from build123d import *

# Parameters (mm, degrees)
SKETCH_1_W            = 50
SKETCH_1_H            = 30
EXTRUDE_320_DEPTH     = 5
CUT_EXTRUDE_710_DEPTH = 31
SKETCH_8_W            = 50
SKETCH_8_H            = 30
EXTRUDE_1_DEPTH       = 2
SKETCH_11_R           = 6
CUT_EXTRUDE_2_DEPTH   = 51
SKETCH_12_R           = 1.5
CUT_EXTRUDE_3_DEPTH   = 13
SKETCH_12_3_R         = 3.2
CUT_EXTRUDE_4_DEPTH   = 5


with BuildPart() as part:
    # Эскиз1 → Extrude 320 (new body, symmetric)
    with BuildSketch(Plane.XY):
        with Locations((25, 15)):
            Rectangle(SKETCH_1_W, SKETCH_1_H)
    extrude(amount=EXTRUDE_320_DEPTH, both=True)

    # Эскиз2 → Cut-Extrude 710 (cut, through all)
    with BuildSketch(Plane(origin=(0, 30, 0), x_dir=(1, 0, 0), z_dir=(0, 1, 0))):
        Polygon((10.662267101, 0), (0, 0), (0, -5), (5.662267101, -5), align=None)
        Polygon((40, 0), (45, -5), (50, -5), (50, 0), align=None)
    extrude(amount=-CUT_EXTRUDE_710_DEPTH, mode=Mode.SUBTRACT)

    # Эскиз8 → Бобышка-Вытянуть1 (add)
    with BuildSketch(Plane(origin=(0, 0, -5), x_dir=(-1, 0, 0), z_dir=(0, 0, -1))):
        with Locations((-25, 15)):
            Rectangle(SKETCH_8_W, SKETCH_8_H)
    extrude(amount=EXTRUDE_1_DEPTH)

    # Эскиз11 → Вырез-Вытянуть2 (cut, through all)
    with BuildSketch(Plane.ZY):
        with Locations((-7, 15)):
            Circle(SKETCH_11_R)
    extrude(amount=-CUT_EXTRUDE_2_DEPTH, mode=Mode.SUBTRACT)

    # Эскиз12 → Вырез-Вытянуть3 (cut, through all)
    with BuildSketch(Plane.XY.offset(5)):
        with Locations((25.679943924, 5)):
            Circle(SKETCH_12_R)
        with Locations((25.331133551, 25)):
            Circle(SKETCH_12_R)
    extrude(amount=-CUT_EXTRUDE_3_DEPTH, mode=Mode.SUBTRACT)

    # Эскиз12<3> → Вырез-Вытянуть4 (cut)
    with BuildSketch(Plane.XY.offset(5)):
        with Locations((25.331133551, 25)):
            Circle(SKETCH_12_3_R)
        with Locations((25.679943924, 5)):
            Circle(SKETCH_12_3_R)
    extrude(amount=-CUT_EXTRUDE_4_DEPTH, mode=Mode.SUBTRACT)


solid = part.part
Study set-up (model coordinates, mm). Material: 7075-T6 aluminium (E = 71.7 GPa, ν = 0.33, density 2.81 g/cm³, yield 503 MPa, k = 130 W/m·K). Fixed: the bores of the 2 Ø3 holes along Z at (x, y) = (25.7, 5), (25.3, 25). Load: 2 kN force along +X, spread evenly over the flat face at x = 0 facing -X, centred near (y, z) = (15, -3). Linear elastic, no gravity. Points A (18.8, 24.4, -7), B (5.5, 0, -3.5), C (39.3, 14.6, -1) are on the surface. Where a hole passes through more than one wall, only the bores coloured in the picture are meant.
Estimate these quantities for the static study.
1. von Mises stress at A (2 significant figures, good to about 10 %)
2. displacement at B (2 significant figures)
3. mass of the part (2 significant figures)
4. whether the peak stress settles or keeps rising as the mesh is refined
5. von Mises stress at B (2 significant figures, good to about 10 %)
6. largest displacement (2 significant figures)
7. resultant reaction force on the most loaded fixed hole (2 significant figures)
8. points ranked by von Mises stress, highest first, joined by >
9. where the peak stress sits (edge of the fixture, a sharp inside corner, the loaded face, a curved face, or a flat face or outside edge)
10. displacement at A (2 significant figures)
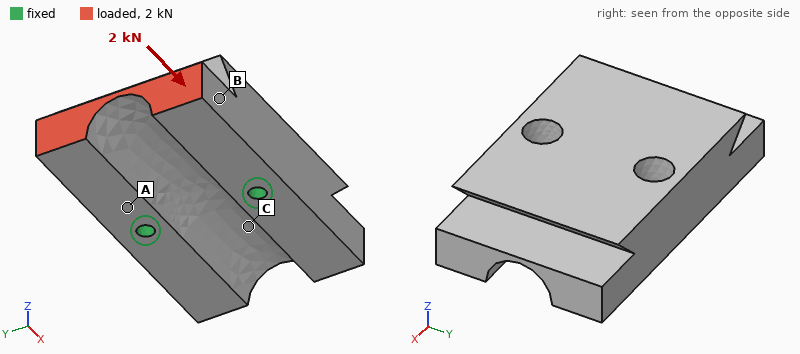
18 MPa
4.4 µm
35 g
keeps rising
13 MPa
6.5 µm
1.0 kN
A > B > C
edge of the fixture
1.5 µm
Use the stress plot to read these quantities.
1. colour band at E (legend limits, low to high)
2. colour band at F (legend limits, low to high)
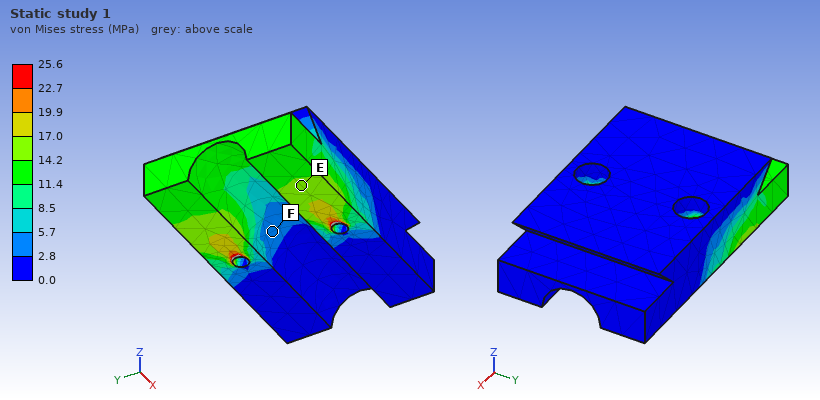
14.2 to 17.0 MPa
2.8 to 5.7 MPa
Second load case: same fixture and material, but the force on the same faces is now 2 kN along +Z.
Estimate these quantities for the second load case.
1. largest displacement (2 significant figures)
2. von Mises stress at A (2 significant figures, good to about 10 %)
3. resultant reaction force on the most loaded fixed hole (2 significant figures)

0.15 mm
110 MPa
1.0 kN
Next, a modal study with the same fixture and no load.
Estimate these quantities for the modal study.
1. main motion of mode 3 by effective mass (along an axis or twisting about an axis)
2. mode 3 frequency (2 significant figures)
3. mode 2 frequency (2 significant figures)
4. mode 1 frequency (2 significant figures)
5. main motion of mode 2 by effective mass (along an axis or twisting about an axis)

along Z
14 kHz
13 kHz
8000 Hz
twisting about Z
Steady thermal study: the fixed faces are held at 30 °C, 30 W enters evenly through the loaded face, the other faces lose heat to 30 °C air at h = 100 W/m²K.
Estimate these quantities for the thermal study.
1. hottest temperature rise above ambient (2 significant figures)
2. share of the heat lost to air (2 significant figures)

30 K
13 %
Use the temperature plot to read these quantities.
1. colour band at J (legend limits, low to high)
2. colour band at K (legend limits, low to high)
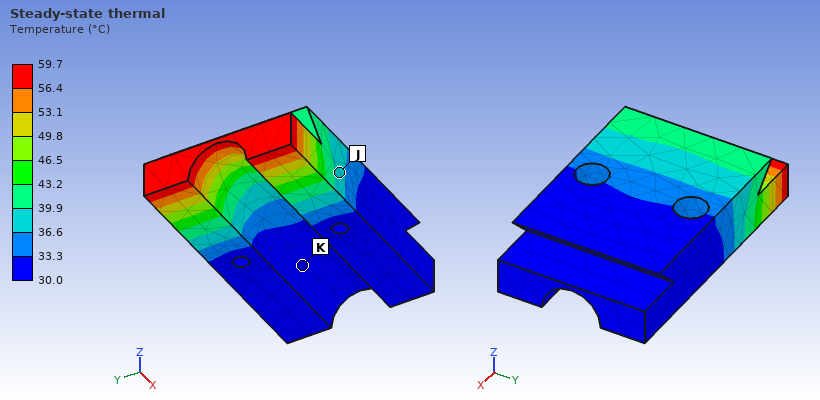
36.6 to 39.9 °C
30.0 to 33.3 °C
